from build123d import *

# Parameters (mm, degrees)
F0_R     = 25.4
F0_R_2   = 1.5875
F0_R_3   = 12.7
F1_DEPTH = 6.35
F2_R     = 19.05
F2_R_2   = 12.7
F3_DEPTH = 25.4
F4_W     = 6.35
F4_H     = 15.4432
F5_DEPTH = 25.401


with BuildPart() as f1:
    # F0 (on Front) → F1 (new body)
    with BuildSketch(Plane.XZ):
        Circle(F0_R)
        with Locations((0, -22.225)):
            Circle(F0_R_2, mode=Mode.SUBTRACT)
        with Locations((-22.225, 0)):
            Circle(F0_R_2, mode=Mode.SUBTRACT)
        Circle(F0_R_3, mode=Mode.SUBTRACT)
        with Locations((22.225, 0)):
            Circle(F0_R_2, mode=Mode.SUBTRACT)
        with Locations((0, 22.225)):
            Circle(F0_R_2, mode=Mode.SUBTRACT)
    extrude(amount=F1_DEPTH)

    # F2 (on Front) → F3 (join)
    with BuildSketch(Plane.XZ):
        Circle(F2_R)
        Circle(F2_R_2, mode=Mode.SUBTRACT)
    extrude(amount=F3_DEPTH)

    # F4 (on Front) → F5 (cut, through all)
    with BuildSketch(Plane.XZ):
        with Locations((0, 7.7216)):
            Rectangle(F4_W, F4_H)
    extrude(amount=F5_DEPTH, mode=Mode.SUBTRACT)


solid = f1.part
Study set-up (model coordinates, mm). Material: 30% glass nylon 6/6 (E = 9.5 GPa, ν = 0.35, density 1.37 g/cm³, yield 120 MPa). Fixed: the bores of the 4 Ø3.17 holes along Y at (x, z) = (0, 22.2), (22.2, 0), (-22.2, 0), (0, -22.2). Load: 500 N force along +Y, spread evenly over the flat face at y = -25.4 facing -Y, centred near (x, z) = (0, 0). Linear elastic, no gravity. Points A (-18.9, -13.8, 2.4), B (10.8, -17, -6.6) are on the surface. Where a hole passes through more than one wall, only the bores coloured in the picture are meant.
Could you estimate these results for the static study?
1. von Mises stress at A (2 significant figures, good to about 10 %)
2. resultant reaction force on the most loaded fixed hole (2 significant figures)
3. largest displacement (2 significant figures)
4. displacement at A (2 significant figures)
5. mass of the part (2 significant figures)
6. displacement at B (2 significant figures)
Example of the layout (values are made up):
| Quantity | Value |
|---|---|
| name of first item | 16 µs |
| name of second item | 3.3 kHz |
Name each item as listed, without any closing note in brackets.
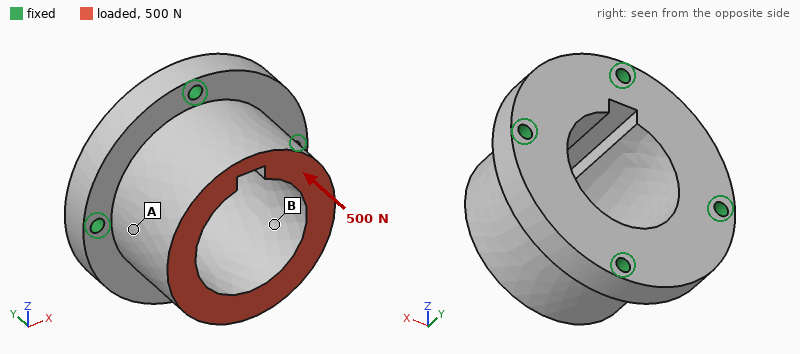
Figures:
| Quantity | Value |
|---|---|
| von Mises stress at A | 1.2 MPa |
| resultant reaction force on the most loaded fixed hole | 130 N |
| largest displacement | 5.8 µm |
| displacement at A | 4.5 µm |
| mass of the part | 29 g |
| displacement at B | 4.7 µm |
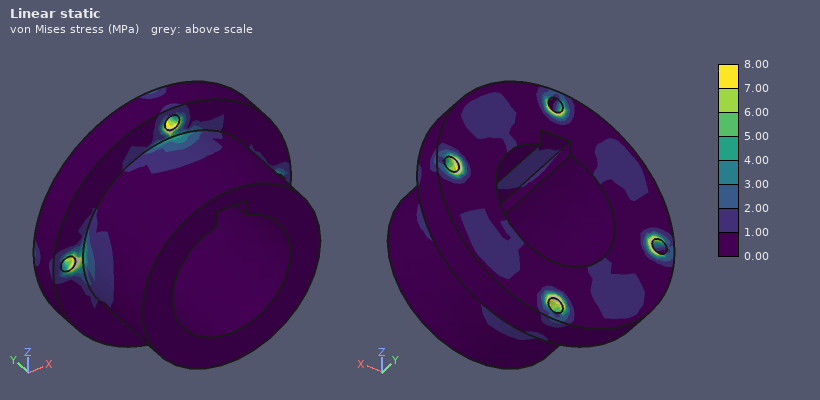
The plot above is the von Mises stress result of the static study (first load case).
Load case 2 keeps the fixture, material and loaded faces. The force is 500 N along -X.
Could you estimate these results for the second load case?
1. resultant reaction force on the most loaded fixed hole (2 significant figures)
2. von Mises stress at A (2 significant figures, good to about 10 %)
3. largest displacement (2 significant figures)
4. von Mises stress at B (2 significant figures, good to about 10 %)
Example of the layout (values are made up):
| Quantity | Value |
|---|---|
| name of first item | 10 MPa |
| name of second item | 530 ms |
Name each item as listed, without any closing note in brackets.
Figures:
| Quantity | Value |
|---|---|
| resultant reaction force on the most loaded fixed hole | 290 N |
| von Mises stress at A | 3.2 MPa |
| largest displacement | 26 µm |
| von Mises stress at B | 3.0 MPa |
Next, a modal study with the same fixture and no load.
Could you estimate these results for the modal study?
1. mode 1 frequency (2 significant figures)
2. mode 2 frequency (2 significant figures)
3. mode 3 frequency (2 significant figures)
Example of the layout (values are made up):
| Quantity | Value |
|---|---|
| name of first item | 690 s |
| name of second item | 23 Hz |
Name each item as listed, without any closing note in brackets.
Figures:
| Quantity | Value |
|---|---|
| mode 1 frequency | 8500 Hz |
| mode 2 frequency | 8600 Hz |
| mode 3 frequency | 9000 Hz |
